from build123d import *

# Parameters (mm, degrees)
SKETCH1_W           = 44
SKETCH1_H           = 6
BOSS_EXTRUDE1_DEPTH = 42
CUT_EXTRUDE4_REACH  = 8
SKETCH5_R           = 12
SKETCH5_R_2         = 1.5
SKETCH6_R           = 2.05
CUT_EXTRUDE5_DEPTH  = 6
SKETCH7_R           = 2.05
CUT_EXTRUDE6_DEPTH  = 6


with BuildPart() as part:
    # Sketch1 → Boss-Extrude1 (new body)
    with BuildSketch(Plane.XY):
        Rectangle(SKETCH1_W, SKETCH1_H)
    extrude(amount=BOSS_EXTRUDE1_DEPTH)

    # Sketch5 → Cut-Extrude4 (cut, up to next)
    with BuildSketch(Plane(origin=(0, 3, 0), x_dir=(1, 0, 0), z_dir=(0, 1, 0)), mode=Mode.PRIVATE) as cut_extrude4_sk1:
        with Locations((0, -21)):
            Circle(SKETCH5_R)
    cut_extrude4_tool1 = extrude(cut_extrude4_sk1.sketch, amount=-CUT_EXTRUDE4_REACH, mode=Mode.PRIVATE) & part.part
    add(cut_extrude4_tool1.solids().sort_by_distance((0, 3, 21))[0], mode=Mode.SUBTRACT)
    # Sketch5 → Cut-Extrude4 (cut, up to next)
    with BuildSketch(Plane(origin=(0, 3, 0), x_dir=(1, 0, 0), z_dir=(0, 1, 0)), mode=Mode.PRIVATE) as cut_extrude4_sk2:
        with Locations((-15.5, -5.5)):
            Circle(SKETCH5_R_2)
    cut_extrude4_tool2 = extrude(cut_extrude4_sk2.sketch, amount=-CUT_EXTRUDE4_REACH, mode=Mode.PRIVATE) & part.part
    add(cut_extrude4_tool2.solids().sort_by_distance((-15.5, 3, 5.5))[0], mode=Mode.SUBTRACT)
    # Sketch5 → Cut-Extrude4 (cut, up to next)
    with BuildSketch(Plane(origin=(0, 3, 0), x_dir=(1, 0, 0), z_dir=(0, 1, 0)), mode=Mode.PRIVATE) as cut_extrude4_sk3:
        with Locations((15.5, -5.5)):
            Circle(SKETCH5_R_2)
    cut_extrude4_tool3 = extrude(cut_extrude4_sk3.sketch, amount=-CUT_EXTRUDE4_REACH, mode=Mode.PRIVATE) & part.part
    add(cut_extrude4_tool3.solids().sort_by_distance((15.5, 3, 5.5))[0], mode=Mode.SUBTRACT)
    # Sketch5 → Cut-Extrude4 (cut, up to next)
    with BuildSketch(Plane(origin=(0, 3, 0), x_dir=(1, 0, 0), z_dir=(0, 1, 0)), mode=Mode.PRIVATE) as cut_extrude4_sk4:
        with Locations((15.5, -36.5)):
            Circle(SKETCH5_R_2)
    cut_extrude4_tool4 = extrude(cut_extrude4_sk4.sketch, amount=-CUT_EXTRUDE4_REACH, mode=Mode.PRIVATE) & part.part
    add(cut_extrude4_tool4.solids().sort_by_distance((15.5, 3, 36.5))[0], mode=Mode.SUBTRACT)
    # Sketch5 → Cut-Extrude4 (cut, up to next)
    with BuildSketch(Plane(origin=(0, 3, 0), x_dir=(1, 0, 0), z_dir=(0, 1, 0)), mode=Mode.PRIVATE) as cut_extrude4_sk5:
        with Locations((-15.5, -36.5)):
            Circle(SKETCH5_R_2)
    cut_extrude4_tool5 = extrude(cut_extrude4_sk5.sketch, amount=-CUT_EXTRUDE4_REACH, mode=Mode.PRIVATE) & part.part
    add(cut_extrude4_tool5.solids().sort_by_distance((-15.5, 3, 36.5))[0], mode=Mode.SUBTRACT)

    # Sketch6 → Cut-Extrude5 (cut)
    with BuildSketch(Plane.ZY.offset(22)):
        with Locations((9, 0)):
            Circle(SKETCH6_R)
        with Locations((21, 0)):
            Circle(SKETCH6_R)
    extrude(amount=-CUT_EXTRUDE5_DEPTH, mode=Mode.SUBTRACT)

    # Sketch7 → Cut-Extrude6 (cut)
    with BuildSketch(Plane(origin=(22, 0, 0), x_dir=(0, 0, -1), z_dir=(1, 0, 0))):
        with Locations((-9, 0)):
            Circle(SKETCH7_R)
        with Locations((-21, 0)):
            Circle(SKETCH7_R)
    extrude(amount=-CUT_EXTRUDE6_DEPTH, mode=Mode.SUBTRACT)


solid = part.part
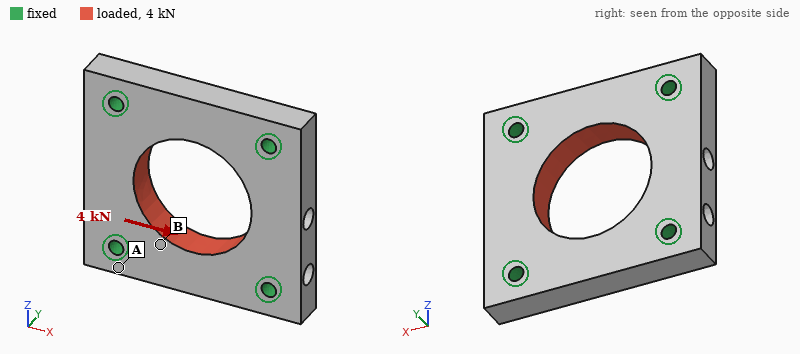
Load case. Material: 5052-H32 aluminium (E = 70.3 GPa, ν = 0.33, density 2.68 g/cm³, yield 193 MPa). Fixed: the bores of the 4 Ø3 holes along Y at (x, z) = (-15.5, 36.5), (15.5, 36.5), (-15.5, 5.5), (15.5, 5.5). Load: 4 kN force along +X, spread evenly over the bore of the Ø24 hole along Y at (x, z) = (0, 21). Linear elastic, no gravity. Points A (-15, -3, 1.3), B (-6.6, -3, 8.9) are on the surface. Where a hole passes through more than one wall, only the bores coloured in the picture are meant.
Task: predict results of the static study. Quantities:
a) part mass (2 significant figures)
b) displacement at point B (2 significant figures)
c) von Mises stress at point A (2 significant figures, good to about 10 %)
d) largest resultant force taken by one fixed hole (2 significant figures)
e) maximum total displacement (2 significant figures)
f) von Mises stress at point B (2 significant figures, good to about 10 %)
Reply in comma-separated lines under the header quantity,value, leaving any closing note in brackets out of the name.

quantity,value
part mass,21 g
displacement at point B,2.6 µm
von Mises stress at point A,6.5 MPa
largest resultant force taken by one fixed hole,1.0 kN
maximum total displacement,7.2 µm
von Mises stress at point B,18 MPa
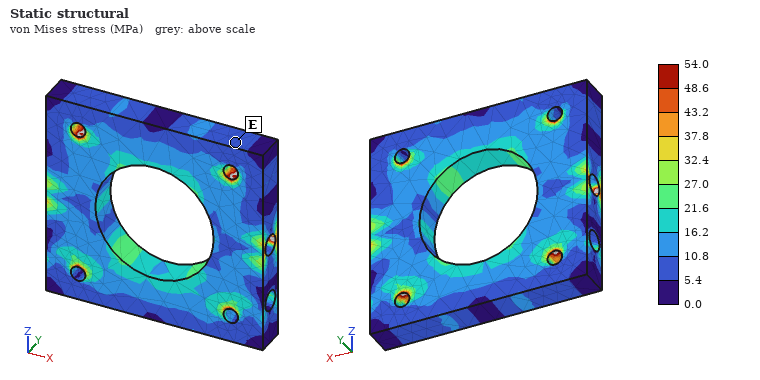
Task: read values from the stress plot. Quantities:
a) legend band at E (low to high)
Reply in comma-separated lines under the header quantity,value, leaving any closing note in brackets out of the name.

quantity,value
legend band at E,5.4 to 10.8 MPa
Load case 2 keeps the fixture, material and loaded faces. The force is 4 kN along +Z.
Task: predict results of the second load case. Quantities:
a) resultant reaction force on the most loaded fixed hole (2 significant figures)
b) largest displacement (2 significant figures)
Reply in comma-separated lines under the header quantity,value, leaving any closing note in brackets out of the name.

quantity,value
resultant reaction force on the most loaded fixed hole,1.1 kN
largest displacement,6.9 µm
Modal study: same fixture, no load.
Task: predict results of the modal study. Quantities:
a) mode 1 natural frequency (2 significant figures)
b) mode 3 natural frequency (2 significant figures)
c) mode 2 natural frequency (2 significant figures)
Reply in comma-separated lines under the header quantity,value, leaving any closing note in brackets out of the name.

quantity,value
mode 1 natural frequency,26 kHz
mode 3 natural frequency,26 kHz
mode 2 natural frequency,26 kHz
